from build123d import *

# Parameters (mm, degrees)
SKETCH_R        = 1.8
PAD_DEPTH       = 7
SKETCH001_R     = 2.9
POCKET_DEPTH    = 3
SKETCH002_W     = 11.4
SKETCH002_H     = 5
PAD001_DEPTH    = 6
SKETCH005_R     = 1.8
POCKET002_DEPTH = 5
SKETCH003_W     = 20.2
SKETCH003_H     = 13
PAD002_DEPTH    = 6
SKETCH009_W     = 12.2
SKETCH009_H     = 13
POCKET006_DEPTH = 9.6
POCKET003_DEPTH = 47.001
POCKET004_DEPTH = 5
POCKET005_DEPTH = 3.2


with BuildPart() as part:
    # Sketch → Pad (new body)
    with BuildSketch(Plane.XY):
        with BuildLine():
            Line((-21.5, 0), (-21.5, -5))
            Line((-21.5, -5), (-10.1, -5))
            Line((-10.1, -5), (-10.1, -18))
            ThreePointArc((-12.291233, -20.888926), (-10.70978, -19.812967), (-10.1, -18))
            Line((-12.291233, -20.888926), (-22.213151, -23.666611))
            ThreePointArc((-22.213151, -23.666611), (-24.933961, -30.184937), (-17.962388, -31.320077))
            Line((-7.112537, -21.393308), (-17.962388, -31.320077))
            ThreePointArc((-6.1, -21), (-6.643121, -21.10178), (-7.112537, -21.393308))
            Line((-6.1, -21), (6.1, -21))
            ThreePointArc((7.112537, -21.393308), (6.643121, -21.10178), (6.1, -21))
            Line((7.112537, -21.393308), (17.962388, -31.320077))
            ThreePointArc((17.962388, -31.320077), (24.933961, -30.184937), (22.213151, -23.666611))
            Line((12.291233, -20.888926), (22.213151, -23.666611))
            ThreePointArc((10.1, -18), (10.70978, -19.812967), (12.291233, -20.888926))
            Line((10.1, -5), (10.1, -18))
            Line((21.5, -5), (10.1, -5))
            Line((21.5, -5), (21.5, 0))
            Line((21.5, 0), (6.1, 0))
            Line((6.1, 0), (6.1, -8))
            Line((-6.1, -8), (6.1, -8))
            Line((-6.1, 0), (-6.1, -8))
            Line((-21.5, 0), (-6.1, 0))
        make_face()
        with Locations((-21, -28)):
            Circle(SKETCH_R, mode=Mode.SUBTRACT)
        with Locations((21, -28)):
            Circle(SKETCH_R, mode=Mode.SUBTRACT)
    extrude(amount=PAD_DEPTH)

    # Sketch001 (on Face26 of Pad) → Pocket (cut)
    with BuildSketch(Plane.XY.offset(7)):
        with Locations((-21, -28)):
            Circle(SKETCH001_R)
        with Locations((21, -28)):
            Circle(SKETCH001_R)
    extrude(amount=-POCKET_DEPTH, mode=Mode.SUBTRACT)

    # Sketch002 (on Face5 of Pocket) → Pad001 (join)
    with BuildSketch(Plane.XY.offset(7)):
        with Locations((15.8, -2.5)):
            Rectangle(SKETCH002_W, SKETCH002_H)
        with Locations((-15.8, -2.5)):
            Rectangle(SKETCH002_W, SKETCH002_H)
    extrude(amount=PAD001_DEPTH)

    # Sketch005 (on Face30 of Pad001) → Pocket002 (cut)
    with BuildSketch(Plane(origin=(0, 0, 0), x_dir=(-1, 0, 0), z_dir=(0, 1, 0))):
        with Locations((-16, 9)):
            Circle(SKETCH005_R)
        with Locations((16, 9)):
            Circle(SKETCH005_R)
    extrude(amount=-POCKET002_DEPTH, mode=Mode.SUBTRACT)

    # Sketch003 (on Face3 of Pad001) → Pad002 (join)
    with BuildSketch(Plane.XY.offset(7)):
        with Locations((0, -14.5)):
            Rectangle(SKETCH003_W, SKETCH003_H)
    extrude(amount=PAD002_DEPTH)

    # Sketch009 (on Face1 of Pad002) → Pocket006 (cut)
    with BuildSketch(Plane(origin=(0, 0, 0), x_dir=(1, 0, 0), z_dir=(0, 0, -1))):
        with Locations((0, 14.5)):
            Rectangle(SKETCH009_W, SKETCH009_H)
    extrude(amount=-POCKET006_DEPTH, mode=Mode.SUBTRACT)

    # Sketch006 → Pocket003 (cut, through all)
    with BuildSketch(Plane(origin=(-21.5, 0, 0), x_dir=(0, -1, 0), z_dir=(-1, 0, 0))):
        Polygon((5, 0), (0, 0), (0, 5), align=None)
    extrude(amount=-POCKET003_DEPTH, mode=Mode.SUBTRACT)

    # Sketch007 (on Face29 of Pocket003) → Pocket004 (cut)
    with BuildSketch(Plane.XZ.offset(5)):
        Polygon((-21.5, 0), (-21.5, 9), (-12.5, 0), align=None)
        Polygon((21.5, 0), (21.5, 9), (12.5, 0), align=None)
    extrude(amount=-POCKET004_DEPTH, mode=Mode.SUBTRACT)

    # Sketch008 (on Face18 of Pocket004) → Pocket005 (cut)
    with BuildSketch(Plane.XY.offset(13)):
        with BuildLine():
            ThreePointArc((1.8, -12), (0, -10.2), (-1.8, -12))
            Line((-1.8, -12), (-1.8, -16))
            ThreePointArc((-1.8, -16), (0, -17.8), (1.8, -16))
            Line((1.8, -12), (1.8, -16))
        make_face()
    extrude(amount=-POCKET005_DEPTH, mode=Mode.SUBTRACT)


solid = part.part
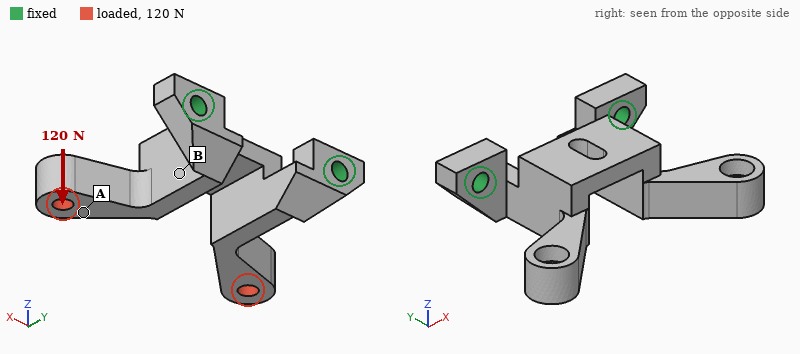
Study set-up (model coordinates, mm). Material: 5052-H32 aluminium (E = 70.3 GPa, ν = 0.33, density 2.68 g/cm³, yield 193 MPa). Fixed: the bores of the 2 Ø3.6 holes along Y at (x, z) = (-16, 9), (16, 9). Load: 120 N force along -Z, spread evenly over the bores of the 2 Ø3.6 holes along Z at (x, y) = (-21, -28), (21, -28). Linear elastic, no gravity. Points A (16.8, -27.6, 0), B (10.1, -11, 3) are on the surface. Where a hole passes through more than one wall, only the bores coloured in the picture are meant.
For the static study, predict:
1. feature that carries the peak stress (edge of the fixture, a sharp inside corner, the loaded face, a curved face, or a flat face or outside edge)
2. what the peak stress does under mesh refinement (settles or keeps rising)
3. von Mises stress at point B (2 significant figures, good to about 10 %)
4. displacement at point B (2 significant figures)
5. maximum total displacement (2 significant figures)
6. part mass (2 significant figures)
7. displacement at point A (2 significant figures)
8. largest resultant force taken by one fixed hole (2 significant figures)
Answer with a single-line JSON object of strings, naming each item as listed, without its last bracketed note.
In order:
{"feature that carries the peak stress": "a sharp inside corner", "what the peak stress does under mesh refinement": "keeps rising", "von Mises stress at point B": "29 MPa", "displacement at point B": "0.038 mm", "maximum total displacement": "0.18 mm", "part mass": "12 g", "displacement at point A": "0.14 mm", "largest resultant force taken by one fixed hole": "75 N"}
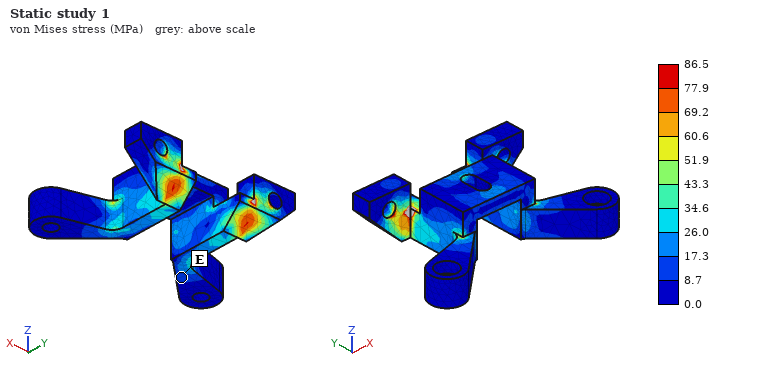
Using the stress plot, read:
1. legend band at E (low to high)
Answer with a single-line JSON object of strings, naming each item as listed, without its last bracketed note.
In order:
{"legend band at E": "8.7 to 17.3 MPa"}
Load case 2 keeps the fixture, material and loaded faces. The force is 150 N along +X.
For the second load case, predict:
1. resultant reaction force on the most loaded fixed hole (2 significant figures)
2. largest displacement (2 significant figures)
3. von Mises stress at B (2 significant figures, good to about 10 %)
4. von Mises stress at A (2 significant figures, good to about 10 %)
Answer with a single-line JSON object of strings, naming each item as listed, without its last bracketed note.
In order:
{"resultant reaction force on the most loaded fixed hole": "160 N", "largest displacement": "0.13 mm", "von Mises stress at B": "26 MPa", "von Mises stress at A": "4.6 MPa"}
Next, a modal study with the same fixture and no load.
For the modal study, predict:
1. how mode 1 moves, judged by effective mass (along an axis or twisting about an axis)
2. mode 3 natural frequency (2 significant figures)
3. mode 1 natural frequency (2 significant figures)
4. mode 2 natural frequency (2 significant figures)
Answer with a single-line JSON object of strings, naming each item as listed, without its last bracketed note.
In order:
{"how mode 1 moves, judged by effective mass": "along Z", "mode 3 natural frequency": "4300 Hz", "mode 1 natural frequency": "2300 Hz", "mode 2 natural frequency": "2800 Hz"}
